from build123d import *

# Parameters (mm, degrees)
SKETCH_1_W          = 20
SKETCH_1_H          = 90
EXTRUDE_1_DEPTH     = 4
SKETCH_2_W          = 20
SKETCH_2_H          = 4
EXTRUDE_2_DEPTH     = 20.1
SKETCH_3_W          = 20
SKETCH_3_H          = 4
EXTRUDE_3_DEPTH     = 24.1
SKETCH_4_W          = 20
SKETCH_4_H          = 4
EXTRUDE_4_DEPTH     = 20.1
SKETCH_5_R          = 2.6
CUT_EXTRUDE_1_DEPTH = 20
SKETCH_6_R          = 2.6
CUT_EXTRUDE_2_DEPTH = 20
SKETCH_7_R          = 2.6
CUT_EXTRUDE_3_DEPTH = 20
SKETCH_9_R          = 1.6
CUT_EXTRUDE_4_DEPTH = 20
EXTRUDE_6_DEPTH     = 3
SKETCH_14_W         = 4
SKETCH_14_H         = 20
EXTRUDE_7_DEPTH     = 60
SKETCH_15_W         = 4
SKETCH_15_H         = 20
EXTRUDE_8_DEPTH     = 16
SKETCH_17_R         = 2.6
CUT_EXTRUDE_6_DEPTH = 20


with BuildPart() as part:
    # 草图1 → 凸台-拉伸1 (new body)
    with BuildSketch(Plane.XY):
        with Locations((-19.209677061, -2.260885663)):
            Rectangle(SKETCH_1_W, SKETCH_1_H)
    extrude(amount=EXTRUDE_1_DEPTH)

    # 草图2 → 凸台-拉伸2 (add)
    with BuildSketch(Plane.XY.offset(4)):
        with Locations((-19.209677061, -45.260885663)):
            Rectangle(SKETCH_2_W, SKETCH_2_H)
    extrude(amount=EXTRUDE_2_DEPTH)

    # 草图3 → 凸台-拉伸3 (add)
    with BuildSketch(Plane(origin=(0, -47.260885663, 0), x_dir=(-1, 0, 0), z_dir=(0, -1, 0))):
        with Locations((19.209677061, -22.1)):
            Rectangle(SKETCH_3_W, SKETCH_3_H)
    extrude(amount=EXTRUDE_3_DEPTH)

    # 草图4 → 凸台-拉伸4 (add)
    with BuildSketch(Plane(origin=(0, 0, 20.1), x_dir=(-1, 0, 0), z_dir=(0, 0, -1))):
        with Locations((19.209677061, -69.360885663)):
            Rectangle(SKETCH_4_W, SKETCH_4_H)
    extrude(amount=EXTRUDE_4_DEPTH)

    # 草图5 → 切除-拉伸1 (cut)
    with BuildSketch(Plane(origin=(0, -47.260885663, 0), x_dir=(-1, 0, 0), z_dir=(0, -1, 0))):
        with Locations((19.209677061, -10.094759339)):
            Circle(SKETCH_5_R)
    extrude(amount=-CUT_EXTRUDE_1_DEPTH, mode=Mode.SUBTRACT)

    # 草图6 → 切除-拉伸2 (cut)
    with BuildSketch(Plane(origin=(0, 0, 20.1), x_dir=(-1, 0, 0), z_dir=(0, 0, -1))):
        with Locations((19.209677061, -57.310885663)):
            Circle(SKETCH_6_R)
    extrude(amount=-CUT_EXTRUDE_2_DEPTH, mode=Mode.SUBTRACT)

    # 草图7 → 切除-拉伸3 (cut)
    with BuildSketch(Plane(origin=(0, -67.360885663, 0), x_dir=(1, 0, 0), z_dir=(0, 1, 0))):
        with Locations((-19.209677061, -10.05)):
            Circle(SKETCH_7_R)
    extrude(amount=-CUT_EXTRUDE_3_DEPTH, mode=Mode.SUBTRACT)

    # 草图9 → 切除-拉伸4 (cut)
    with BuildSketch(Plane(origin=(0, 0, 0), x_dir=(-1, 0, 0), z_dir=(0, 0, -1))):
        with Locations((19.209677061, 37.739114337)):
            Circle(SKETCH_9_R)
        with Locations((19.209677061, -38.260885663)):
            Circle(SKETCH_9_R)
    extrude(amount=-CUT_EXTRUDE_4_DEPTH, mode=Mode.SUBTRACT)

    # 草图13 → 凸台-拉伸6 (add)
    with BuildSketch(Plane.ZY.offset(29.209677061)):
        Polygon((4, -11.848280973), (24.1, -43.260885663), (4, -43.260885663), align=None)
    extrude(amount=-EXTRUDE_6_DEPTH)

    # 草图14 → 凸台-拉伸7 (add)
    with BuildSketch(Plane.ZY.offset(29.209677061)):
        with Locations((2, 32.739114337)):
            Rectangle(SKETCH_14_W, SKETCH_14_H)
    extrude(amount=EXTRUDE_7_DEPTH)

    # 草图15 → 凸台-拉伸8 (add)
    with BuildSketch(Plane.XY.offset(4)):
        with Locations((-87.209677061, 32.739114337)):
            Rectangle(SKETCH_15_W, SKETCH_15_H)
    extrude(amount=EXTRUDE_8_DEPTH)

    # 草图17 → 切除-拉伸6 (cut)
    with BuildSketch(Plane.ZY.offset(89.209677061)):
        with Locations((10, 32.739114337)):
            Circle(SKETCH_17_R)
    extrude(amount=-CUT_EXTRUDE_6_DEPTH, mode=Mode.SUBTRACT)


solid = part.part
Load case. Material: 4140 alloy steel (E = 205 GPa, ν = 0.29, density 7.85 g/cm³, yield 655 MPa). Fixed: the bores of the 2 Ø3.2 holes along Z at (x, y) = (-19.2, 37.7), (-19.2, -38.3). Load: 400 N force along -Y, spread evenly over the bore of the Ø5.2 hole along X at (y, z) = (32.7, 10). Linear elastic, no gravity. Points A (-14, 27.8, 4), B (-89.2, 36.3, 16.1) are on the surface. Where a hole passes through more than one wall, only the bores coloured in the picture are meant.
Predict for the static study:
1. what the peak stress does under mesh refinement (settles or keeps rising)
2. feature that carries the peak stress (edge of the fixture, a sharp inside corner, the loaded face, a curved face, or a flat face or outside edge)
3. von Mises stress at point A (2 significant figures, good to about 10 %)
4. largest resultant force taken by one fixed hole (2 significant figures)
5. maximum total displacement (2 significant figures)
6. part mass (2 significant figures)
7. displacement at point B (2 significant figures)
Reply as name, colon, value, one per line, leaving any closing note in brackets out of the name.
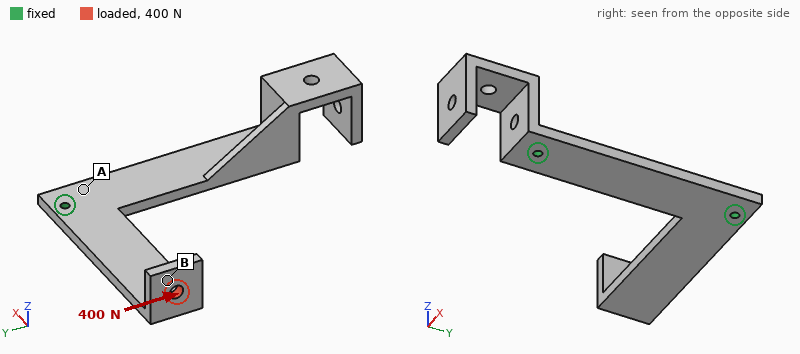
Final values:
what the peak stress does under mesh refinement: keeps rising
feature that carries the peak stress: edge of the fixture
von Mises stress at point A: 25 MPa
largest resultant force taken by one fixed hole: 390 N
maximum total displacement: 0.25 mm
part mass: 150 g
displacement at point B: 0.21 mm
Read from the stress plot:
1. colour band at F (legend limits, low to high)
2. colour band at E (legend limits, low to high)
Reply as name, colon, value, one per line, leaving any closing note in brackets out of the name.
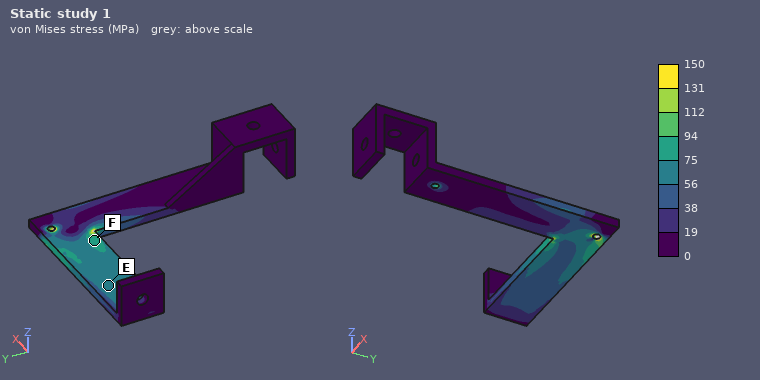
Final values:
colour band at F: 75 to 94 MPa
colour band at E: 56 to 75 MPa
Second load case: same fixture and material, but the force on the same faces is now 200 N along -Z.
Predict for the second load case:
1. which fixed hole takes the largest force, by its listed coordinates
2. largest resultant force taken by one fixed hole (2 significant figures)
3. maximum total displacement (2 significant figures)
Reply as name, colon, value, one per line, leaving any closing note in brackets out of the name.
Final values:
which fixed hole takes the largest force, by its listed coordinates: (-19.2, 37.7)
largest resultant force taken by one fixed hole: 210 N
maximum total displacement: 1.1 mm
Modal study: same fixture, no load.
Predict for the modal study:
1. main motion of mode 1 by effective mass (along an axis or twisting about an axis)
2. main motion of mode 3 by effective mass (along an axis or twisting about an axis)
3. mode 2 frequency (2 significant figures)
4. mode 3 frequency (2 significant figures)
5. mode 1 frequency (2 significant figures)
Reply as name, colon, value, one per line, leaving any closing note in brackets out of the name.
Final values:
main motion of mode 1 by effective mass: along Z
main motion of mode 3 by effective mass: along Y
mode 2 frequency: 1500 Hz
mode 3 frequency: 1800 Hz
mode 1 frequency: 490 Hz
